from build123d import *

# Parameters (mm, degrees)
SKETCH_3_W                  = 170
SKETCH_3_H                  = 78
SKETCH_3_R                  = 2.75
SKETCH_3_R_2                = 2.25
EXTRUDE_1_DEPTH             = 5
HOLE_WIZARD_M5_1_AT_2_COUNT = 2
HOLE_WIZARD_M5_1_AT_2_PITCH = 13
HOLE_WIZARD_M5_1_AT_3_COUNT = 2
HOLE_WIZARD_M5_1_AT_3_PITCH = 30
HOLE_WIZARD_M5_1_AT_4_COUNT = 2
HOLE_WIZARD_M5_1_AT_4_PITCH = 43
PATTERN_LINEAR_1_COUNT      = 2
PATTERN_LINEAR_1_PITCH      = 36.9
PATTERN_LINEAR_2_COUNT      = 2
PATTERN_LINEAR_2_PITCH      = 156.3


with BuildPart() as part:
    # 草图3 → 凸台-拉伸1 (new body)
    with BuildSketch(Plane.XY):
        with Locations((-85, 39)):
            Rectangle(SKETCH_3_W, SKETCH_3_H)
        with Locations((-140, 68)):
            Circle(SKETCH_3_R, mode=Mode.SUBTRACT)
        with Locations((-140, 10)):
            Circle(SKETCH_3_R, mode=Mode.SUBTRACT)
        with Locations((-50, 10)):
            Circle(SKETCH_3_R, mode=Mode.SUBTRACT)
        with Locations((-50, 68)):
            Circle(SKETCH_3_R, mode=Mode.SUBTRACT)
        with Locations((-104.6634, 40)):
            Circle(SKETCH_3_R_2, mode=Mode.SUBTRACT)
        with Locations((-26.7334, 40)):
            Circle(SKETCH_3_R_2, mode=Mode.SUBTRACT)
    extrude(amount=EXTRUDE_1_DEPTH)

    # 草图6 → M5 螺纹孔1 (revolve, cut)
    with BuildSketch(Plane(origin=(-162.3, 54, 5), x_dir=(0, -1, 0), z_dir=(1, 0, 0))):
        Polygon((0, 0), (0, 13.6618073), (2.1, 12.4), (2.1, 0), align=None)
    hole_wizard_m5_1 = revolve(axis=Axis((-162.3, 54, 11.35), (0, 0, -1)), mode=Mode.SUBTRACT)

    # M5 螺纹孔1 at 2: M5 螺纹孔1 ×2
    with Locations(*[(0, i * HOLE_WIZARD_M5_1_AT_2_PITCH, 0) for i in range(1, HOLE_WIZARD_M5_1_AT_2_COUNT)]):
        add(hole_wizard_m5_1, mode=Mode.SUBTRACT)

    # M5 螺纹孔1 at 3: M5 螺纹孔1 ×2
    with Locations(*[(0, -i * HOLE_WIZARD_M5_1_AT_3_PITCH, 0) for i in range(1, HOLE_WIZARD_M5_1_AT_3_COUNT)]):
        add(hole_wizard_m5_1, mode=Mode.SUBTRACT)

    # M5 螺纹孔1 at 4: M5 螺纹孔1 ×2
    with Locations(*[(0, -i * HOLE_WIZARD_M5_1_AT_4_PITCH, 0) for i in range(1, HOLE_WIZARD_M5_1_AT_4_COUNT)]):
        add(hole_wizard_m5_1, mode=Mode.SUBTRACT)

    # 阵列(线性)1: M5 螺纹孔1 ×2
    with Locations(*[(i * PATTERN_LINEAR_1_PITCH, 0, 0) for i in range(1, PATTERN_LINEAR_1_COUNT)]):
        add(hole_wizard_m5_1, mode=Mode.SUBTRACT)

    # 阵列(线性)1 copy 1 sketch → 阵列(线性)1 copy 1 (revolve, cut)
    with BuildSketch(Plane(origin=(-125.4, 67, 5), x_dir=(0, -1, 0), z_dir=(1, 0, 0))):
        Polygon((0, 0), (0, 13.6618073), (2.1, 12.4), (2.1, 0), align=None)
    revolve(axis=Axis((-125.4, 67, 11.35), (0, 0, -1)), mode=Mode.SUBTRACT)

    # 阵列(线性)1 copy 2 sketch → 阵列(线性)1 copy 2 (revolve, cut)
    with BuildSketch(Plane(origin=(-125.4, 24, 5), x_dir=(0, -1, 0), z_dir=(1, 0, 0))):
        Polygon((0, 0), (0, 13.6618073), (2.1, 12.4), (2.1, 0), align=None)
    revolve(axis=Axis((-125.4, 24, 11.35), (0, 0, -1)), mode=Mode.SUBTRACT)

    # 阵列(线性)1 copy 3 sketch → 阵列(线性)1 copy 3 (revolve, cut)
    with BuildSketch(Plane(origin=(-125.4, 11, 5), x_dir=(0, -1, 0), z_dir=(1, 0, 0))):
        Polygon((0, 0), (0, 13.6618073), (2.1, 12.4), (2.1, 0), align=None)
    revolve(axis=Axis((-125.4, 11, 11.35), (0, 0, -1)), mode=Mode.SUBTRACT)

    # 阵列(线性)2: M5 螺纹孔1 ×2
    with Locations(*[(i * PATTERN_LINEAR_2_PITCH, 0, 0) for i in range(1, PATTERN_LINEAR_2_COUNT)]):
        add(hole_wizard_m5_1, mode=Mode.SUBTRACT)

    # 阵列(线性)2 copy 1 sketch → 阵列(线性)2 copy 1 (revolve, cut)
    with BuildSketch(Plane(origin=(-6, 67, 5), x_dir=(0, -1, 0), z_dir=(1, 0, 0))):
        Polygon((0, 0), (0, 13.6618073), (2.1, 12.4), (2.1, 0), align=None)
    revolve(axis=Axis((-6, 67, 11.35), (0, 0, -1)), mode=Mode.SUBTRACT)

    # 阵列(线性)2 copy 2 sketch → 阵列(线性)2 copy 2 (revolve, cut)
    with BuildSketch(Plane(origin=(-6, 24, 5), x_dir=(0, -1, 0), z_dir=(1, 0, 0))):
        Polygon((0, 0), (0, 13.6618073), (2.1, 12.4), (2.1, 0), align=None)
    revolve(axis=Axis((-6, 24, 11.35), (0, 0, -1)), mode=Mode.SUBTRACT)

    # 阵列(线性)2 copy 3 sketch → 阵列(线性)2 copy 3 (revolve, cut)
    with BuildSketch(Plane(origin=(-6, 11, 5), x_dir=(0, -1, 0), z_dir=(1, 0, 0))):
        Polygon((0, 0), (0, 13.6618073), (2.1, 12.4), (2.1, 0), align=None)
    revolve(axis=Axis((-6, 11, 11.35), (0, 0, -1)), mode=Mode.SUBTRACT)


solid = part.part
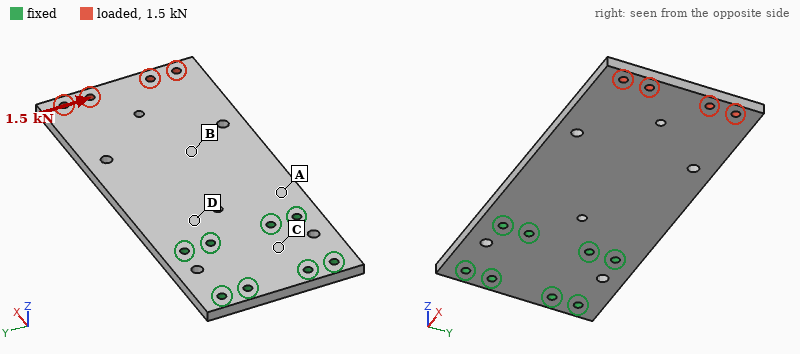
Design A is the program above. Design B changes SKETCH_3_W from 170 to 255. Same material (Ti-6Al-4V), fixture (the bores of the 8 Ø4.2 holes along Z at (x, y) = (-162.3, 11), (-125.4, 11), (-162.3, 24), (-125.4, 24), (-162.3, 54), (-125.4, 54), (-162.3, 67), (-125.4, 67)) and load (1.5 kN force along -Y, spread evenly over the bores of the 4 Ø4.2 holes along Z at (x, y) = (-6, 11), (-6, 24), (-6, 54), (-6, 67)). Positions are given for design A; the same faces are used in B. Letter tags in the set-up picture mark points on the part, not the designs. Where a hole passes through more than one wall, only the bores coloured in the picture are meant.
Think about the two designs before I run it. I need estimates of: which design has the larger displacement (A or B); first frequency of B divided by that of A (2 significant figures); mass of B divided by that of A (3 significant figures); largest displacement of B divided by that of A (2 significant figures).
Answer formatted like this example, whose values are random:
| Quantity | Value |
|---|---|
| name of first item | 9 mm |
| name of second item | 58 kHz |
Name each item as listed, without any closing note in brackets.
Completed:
| Quantity | Value |
|---|---|
| which design has the larger displacement | B |
| first frequency of B divided by that of A | 0.55 |
| mass of B divided by that of A | 1.51 |
| largest displacement of B divided by that of A | 1.3 |
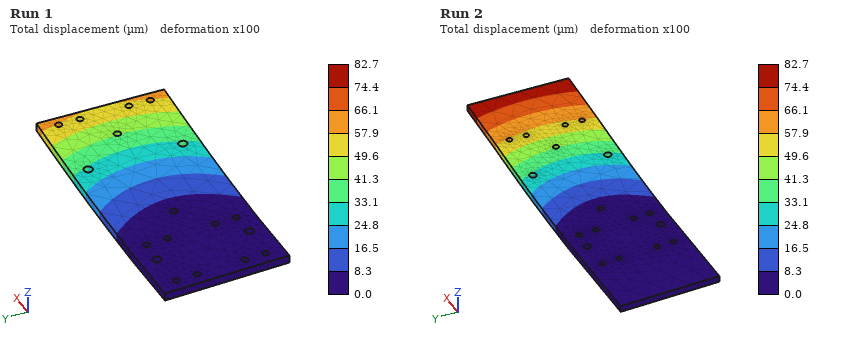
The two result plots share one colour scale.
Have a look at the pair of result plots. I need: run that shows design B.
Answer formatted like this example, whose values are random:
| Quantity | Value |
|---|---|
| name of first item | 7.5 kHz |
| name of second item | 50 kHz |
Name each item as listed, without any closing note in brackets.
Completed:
| Quantity | Value |
|---|---|
| run that shows design B | Run 2 |
